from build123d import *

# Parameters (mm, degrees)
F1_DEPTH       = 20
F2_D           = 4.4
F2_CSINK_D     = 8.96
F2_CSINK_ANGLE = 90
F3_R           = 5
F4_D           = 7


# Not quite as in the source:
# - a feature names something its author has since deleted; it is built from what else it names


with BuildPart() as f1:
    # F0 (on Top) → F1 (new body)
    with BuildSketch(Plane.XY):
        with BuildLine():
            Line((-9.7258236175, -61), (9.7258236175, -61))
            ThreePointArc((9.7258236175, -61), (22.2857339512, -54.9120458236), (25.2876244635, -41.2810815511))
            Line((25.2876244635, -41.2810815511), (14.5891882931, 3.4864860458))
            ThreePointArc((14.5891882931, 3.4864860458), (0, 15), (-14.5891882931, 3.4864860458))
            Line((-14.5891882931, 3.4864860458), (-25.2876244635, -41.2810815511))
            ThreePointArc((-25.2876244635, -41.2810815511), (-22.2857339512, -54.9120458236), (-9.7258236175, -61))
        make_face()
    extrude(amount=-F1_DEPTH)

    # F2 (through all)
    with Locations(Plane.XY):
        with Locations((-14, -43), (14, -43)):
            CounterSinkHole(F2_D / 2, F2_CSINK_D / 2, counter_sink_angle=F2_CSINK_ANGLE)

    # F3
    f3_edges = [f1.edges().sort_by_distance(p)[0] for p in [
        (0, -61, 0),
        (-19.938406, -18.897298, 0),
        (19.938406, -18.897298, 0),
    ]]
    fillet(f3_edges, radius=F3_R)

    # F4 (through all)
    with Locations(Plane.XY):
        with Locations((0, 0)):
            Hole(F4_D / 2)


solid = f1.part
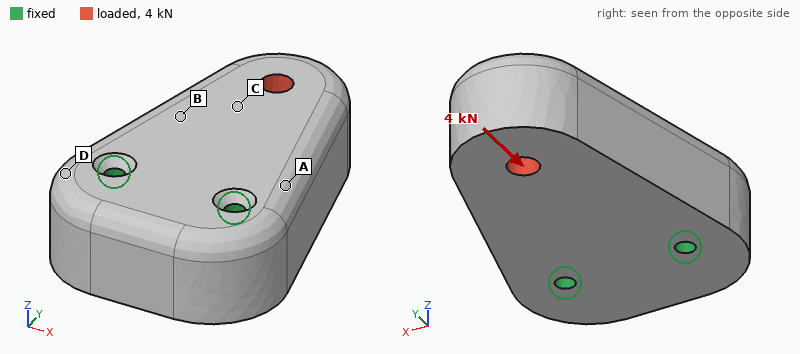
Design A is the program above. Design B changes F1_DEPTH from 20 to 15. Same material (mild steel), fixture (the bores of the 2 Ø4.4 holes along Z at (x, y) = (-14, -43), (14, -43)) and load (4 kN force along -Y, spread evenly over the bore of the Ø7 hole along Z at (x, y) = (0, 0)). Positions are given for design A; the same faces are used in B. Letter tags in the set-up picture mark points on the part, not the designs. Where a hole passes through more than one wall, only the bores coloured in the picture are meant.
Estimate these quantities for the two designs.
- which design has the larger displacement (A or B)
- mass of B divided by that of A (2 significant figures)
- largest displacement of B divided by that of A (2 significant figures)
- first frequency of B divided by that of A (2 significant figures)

B
0.74
1.4
0.78
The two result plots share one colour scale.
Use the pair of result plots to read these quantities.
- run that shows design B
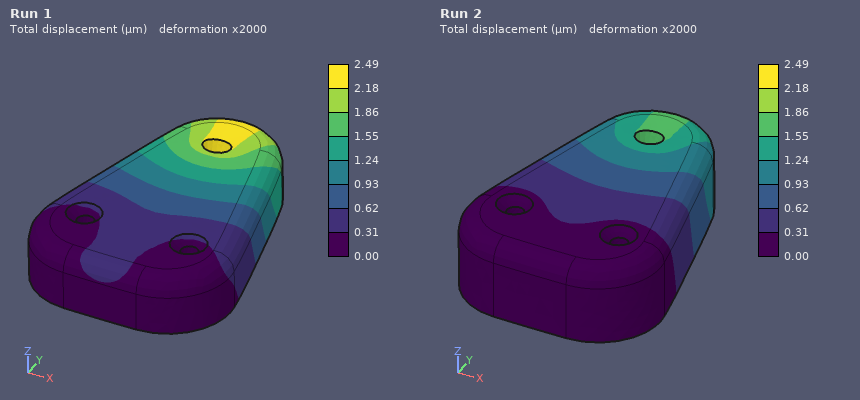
Run 1
